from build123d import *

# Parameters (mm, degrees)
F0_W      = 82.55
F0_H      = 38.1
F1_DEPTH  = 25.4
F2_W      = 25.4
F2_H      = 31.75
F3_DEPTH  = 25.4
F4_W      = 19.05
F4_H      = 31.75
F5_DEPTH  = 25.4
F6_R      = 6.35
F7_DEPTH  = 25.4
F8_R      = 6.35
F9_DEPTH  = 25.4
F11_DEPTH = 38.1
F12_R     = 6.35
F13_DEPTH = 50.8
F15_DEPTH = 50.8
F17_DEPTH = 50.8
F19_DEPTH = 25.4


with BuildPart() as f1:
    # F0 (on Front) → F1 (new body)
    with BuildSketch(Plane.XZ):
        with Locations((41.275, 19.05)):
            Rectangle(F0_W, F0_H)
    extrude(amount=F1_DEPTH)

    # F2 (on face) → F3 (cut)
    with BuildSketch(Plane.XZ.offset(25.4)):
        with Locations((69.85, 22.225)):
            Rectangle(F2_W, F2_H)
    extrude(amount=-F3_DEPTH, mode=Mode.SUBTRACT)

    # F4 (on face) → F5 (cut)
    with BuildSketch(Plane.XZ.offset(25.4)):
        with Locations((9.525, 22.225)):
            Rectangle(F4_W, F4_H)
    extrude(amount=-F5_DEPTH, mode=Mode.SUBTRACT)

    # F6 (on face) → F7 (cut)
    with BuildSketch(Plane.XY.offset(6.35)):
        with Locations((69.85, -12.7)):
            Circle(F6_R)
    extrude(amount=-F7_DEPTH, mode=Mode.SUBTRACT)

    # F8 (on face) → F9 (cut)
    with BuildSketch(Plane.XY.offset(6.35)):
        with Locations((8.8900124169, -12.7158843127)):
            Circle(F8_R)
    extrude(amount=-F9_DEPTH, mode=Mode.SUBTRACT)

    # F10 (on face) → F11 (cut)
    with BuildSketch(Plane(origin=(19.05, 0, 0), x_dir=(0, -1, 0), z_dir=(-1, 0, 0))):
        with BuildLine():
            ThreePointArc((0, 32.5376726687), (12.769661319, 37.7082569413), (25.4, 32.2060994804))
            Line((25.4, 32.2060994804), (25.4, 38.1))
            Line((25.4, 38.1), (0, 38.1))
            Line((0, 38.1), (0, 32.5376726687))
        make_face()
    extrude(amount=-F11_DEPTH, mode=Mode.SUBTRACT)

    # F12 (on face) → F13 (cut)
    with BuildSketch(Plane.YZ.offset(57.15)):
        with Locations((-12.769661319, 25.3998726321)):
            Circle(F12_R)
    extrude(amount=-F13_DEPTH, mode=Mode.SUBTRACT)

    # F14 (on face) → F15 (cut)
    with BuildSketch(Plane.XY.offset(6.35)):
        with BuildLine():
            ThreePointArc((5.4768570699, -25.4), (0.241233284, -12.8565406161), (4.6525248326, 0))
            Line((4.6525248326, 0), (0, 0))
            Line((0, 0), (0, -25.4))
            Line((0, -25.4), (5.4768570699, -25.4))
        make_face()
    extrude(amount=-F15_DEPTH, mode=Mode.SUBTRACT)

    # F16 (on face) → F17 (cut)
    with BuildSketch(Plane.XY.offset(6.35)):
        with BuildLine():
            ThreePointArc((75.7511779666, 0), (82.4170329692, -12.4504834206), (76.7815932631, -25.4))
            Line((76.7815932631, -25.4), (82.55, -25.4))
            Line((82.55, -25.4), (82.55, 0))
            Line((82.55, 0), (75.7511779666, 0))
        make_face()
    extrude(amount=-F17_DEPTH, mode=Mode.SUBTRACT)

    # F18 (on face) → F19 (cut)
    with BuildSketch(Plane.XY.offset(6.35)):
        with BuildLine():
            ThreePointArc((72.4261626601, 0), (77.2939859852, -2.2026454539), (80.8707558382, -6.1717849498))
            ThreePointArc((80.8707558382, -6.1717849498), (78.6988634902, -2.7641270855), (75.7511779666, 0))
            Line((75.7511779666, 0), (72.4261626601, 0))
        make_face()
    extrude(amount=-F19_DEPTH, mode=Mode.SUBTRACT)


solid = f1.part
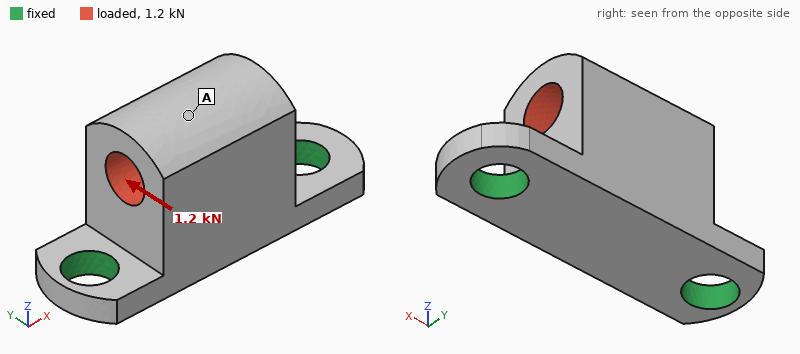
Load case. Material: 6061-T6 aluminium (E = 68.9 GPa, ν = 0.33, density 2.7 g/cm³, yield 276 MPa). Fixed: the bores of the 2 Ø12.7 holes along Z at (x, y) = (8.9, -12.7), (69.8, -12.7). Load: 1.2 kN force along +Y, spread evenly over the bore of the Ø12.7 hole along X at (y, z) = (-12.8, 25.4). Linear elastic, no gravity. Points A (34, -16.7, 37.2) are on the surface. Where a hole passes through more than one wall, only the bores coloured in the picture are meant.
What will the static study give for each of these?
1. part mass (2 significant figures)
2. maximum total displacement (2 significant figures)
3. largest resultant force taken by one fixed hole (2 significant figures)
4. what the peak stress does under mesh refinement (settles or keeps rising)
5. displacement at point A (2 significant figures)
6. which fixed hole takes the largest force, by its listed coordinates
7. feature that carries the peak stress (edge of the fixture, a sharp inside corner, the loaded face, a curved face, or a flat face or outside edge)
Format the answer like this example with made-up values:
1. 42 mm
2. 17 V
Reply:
1. 94 g
2. 56 µm
3. 650 N
4. keeps rising
5. 55 µm
6. (8.9, -12.7)
7. edge of the fixture
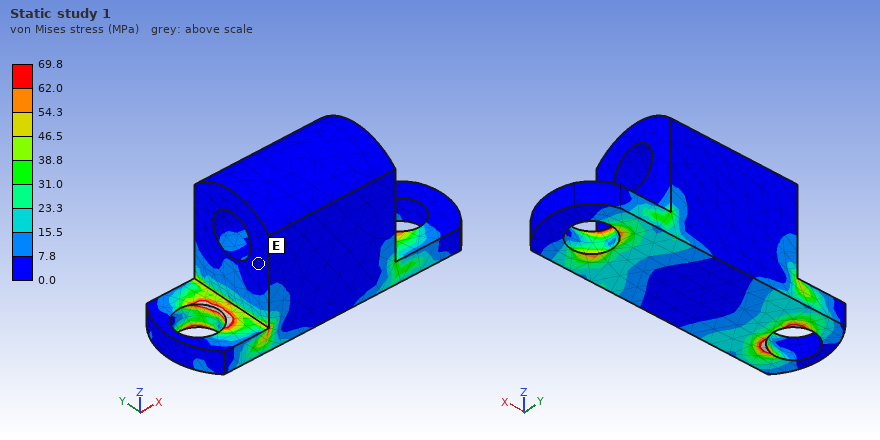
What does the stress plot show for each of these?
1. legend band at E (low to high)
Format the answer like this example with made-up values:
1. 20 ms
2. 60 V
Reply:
1. 0.0 to 7.8 MPa
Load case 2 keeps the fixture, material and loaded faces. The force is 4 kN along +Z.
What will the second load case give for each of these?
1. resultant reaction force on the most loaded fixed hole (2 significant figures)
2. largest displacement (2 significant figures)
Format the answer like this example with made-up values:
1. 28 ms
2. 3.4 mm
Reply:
1. 2.3 kN
2. 16 µm
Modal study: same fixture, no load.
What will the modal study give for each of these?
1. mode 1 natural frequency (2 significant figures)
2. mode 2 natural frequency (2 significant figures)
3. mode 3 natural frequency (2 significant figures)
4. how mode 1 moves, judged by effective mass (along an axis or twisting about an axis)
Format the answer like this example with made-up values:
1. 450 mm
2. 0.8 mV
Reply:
1. 3800 Hz
2. 9500 Hz
3. 11 kHz
4. along Y
